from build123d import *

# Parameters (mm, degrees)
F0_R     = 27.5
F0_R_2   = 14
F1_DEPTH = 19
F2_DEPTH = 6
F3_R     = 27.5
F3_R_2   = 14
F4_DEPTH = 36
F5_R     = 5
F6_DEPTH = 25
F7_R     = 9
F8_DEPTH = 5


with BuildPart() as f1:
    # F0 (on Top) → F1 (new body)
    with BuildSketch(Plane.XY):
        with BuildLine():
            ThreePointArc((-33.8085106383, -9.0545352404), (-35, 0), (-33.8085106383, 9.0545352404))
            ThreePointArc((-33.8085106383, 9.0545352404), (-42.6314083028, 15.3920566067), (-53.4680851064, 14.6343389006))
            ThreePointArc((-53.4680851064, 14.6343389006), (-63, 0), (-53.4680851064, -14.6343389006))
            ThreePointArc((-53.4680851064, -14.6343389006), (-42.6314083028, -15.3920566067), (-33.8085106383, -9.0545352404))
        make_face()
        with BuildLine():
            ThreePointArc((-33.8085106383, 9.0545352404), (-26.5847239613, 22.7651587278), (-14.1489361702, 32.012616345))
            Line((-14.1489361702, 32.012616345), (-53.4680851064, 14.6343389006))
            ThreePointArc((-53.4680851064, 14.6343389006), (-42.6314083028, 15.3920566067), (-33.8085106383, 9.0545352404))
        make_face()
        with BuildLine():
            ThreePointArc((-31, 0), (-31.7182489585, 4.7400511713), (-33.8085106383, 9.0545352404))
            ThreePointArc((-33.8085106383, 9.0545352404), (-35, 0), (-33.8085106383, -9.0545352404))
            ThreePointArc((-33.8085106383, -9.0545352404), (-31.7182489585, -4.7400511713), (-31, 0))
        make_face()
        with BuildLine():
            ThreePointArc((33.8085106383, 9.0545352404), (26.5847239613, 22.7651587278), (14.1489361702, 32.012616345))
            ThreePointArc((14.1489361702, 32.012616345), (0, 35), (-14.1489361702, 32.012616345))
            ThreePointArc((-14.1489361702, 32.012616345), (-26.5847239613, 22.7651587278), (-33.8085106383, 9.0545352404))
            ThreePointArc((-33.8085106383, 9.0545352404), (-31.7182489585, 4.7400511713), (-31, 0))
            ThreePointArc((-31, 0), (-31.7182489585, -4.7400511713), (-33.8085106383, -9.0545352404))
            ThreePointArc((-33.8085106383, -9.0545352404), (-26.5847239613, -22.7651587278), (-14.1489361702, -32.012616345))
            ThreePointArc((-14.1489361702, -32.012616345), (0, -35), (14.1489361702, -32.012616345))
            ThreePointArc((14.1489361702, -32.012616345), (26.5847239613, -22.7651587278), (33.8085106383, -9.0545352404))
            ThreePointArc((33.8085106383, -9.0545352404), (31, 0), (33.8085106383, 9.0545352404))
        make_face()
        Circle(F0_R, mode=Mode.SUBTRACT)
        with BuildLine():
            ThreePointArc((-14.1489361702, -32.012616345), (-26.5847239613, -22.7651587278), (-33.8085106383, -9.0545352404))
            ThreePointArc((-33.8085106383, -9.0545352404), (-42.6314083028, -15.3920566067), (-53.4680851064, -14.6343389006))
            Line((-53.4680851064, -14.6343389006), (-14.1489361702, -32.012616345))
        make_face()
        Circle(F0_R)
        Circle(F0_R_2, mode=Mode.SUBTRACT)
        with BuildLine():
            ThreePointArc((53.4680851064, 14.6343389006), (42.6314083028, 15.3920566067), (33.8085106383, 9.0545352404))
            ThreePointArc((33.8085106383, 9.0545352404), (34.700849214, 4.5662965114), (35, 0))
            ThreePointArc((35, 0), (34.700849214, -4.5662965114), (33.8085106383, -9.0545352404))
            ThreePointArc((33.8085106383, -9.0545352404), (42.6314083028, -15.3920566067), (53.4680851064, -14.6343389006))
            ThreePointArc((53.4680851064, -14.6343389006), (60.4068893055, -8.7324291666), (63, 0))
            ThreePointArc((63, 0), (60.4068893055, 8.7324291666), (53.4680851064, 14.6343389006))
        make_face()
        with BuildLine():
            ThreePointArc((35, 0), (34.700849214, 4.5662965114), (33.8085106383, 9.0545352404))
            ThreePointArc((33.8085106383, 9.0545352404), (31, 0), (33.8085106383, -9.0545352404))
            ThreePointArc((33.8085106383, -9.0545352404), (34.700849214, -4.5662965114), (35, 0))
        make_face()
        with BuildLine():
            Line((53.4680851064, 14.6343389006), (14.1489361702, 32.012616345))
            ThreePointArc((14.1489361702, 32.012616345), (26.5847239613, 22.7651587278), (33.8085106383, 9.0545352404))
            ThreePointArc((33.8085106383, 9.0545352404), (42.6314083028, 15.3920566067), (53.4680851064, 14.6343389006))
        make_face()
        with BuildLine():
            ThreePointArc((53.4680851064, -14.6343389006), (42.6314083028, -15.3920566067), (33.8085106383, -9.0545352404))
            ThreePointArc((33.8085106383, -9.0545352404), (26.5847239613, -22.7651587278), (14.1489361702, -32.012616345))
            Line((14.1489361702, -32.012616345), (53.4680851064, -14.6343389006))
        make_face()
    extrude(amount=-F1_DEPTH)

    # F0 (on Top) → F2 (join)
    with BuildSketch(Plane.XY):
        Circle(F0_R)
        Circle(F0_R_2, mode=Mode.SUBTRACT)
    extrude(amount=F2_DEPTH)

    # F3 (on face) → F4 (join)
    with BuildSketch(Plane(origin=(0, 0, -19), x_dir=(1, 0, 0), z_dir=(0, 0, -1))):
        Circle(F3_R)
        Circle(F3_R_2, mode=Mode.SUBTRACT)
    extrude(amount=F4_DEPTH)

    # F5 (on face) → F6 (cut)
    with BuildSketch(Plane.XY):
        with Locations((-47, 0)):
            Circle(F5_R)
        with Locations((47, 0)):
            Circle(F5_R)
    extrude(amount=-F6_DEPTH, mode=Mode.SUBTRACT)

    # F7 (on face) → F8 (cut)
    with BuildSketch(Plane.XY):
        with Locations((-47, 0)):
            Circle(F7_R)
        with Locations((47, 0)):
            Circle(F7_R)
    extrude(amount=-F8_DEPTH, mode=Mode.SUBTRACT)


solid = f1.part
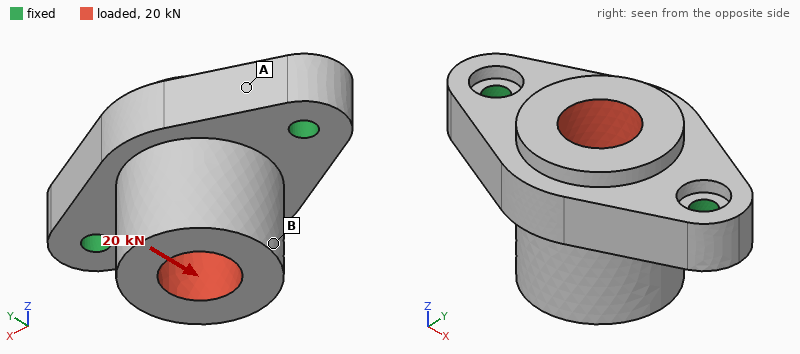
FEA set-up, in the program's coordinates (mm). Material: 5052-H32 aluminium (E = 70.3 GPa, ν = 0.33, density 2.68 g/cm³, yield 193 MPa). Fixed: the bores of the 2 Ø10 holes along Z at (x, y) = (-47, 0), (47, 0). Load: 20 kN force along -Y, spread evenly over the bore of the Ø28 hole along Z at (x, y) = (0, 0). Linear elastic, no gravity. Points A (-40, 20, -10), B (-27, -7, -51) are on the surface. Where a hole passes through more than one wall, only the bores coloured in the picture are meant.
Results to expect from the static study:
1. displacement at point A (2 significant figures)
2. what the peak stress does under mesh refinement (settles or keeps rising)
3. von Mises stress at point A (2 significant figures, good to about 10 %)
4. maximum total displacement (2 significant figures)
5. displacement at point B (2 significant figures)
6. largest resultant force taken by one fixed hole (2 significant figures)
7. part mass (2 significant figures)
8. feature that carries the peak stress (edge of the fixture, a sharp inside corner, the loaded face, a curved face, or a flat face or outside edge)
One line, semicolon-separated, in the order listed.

0.029 mm; keeps rising; 46 MPa; 0.15 mm; 0.12 mm; 10 kN; 460 g; edge of the fixture
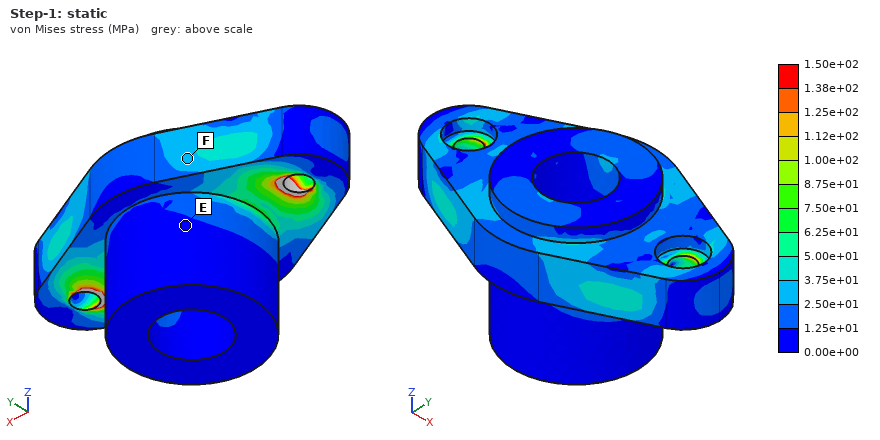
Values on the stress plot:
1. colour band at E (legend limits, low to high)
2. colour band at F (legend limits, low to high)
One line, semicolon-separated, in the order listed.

0.00e+00 to 1.25e+01 MPa; 2.50e+01 to 3.75e+01 MPa
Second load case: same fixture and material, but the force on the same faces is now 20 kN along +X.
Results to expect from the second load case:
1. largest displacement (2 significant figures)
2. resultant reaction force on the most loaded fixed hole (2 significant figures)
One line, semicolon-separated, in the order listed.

34 µm; 11 kN
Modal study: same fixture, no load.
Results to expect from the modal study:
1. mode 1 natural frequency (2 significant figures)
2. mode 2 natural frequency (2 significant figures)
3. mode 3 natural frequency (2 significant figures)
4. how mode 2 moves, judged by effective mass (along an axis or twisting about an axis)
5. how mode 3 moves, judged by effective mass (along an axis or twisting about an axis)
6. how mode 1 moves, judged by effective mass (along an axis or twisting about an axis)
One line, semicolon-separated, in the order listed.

3300 Hz; 6000 Hz; 8100 Hz; along Z; along X; along Y
